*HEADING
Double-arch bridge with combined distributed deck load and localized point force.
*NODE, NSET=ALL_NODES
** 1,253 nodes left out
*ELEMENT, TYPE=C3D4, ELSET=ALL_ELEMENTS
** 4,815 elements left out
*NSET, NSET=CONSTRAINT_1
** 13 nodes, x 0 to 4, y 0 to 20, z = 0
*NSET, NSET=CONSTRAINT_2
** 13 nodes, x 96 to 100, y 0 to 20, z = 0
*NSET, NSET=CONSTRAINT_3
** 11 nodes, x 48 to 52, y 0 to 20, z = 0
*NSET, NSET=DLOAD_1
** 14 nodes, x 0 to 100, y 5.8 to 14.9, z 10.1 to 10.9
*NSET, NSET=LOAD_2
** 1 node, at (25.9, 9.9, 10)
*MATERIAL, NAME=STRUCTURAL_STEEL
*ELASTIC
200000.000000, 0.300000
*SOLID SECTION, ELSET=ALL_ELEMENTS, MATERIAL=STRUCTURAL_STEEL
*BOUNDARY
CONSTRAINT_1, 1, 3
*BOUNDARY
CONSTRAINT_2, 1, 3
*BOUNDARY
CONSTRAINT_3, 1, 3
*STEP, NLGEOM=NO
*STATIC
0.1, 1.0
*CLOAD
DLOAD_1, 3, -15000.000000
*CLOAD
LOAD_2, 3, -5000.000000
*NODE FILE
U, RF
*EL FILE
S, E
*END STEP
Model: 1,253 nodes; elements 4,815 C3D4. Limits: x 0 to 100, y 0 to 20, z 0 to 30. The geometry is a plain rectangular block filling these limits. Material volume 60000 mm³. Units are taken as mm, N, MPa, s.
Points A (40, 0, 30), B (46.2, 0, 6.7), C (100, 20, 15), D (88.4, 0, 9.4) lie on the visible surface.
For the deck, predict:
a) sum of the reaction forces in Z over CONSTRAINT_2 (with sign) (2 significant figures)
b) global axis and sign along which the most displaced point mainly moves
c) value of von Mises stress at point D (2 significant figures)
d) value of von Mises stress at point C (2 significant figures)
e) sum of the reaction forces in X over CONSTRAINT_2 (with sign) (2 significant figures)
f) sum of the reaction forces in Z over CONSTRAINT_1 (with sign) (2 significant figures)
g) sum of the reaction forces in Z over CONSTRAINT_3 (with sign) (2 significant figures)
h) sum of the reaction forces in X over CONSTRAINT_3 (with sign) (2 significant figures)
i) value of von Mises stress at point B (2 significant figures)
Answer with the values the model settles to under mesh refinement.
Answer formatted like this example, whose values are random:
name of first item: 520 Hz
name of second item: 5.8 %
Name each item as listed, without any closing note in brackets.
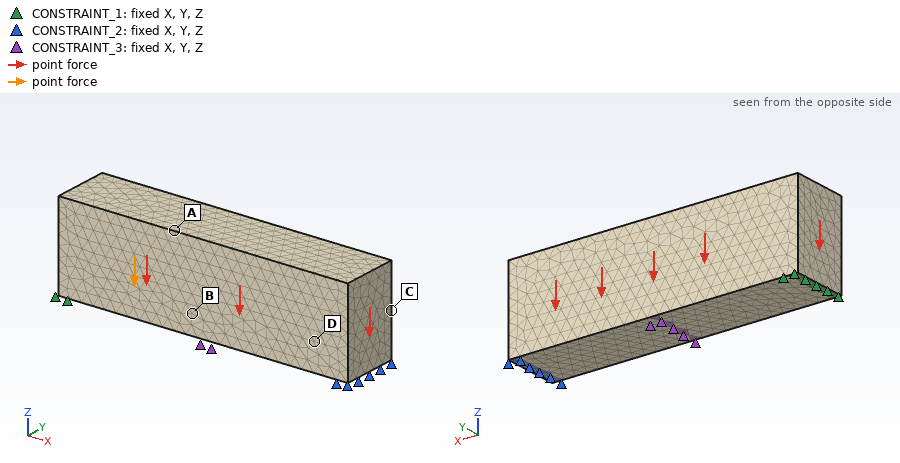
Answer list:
sum of the reaction forces in Z over CONSTRAINT_2 (with sign): 72000 N
global axis and sign along which the most displaced point mainly moves: -Z
value of von Mises stress at point D: 150 MPa
value of von Mises stress at point C: 180 MPa
sum of the reaction forces in X over CONSTRAINT_2 (with sign): -14000 N
sum of the reaction forces in Z over CONSTRAINT_1 (with sign): 72000 N
sum of the reaction forces in Z over CONSTRAINT_3 (with sign): 71000 N
sum of the reaction forces in X over CONSTRAINT_3 (with sign): 3300 N
value of von Mises stress at point B: 200 MPa
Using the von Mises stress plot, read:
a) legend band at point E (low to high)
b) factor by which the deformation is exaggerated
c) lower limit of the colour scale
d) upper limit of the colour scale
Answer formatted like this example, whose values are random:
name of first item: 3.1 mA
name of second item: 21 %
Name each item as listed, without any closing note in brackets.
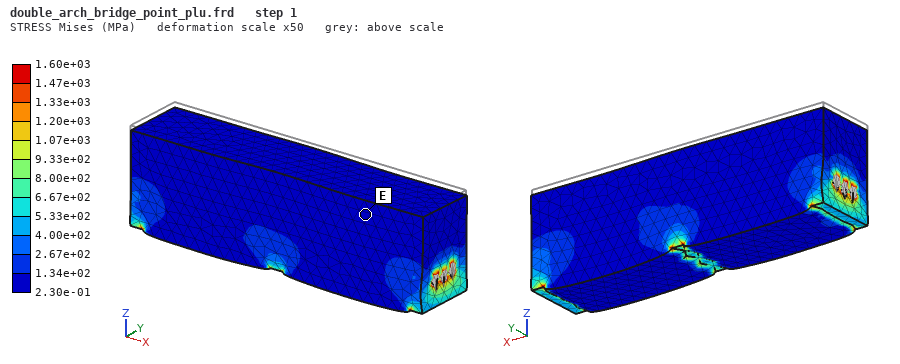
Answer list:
legend band at point E: 2.30e-01 to 1.34e+02 MPa
factor by which the deformation is exaggerated: 50
lower limit of the colour scale: 2.30e-01 MPa
upper limit of the colour scale: 1.60e+03 MPa
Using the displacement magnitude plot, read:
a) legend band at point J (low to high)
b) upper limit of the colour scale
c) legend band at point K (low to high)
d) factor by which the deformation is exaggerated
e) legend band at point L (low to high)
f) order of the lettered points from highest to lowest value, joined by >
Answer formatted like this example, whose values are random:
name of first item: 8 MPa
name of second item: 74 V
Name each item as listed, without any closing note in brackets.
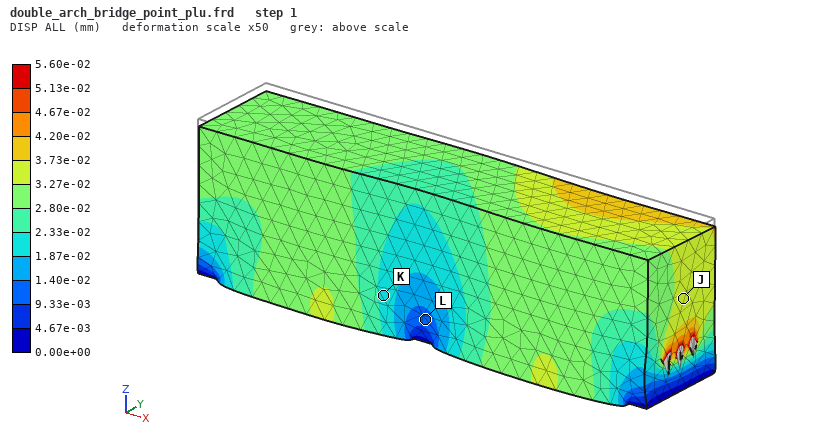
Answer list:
legend band at point J: 3.27e-02 to 3.73e-02 mm
upper limit of the colour scale: 5.60e-02 mm
legend band at point K: 1.87e-02 to 2.33e-02 mm
factor by which the deformation is exaggerated: 50
legend band at point L: 9.33e-03 to 1.40e-02 mm
order of the lettered points from highest to lowest value, joined by >: J > K > L
